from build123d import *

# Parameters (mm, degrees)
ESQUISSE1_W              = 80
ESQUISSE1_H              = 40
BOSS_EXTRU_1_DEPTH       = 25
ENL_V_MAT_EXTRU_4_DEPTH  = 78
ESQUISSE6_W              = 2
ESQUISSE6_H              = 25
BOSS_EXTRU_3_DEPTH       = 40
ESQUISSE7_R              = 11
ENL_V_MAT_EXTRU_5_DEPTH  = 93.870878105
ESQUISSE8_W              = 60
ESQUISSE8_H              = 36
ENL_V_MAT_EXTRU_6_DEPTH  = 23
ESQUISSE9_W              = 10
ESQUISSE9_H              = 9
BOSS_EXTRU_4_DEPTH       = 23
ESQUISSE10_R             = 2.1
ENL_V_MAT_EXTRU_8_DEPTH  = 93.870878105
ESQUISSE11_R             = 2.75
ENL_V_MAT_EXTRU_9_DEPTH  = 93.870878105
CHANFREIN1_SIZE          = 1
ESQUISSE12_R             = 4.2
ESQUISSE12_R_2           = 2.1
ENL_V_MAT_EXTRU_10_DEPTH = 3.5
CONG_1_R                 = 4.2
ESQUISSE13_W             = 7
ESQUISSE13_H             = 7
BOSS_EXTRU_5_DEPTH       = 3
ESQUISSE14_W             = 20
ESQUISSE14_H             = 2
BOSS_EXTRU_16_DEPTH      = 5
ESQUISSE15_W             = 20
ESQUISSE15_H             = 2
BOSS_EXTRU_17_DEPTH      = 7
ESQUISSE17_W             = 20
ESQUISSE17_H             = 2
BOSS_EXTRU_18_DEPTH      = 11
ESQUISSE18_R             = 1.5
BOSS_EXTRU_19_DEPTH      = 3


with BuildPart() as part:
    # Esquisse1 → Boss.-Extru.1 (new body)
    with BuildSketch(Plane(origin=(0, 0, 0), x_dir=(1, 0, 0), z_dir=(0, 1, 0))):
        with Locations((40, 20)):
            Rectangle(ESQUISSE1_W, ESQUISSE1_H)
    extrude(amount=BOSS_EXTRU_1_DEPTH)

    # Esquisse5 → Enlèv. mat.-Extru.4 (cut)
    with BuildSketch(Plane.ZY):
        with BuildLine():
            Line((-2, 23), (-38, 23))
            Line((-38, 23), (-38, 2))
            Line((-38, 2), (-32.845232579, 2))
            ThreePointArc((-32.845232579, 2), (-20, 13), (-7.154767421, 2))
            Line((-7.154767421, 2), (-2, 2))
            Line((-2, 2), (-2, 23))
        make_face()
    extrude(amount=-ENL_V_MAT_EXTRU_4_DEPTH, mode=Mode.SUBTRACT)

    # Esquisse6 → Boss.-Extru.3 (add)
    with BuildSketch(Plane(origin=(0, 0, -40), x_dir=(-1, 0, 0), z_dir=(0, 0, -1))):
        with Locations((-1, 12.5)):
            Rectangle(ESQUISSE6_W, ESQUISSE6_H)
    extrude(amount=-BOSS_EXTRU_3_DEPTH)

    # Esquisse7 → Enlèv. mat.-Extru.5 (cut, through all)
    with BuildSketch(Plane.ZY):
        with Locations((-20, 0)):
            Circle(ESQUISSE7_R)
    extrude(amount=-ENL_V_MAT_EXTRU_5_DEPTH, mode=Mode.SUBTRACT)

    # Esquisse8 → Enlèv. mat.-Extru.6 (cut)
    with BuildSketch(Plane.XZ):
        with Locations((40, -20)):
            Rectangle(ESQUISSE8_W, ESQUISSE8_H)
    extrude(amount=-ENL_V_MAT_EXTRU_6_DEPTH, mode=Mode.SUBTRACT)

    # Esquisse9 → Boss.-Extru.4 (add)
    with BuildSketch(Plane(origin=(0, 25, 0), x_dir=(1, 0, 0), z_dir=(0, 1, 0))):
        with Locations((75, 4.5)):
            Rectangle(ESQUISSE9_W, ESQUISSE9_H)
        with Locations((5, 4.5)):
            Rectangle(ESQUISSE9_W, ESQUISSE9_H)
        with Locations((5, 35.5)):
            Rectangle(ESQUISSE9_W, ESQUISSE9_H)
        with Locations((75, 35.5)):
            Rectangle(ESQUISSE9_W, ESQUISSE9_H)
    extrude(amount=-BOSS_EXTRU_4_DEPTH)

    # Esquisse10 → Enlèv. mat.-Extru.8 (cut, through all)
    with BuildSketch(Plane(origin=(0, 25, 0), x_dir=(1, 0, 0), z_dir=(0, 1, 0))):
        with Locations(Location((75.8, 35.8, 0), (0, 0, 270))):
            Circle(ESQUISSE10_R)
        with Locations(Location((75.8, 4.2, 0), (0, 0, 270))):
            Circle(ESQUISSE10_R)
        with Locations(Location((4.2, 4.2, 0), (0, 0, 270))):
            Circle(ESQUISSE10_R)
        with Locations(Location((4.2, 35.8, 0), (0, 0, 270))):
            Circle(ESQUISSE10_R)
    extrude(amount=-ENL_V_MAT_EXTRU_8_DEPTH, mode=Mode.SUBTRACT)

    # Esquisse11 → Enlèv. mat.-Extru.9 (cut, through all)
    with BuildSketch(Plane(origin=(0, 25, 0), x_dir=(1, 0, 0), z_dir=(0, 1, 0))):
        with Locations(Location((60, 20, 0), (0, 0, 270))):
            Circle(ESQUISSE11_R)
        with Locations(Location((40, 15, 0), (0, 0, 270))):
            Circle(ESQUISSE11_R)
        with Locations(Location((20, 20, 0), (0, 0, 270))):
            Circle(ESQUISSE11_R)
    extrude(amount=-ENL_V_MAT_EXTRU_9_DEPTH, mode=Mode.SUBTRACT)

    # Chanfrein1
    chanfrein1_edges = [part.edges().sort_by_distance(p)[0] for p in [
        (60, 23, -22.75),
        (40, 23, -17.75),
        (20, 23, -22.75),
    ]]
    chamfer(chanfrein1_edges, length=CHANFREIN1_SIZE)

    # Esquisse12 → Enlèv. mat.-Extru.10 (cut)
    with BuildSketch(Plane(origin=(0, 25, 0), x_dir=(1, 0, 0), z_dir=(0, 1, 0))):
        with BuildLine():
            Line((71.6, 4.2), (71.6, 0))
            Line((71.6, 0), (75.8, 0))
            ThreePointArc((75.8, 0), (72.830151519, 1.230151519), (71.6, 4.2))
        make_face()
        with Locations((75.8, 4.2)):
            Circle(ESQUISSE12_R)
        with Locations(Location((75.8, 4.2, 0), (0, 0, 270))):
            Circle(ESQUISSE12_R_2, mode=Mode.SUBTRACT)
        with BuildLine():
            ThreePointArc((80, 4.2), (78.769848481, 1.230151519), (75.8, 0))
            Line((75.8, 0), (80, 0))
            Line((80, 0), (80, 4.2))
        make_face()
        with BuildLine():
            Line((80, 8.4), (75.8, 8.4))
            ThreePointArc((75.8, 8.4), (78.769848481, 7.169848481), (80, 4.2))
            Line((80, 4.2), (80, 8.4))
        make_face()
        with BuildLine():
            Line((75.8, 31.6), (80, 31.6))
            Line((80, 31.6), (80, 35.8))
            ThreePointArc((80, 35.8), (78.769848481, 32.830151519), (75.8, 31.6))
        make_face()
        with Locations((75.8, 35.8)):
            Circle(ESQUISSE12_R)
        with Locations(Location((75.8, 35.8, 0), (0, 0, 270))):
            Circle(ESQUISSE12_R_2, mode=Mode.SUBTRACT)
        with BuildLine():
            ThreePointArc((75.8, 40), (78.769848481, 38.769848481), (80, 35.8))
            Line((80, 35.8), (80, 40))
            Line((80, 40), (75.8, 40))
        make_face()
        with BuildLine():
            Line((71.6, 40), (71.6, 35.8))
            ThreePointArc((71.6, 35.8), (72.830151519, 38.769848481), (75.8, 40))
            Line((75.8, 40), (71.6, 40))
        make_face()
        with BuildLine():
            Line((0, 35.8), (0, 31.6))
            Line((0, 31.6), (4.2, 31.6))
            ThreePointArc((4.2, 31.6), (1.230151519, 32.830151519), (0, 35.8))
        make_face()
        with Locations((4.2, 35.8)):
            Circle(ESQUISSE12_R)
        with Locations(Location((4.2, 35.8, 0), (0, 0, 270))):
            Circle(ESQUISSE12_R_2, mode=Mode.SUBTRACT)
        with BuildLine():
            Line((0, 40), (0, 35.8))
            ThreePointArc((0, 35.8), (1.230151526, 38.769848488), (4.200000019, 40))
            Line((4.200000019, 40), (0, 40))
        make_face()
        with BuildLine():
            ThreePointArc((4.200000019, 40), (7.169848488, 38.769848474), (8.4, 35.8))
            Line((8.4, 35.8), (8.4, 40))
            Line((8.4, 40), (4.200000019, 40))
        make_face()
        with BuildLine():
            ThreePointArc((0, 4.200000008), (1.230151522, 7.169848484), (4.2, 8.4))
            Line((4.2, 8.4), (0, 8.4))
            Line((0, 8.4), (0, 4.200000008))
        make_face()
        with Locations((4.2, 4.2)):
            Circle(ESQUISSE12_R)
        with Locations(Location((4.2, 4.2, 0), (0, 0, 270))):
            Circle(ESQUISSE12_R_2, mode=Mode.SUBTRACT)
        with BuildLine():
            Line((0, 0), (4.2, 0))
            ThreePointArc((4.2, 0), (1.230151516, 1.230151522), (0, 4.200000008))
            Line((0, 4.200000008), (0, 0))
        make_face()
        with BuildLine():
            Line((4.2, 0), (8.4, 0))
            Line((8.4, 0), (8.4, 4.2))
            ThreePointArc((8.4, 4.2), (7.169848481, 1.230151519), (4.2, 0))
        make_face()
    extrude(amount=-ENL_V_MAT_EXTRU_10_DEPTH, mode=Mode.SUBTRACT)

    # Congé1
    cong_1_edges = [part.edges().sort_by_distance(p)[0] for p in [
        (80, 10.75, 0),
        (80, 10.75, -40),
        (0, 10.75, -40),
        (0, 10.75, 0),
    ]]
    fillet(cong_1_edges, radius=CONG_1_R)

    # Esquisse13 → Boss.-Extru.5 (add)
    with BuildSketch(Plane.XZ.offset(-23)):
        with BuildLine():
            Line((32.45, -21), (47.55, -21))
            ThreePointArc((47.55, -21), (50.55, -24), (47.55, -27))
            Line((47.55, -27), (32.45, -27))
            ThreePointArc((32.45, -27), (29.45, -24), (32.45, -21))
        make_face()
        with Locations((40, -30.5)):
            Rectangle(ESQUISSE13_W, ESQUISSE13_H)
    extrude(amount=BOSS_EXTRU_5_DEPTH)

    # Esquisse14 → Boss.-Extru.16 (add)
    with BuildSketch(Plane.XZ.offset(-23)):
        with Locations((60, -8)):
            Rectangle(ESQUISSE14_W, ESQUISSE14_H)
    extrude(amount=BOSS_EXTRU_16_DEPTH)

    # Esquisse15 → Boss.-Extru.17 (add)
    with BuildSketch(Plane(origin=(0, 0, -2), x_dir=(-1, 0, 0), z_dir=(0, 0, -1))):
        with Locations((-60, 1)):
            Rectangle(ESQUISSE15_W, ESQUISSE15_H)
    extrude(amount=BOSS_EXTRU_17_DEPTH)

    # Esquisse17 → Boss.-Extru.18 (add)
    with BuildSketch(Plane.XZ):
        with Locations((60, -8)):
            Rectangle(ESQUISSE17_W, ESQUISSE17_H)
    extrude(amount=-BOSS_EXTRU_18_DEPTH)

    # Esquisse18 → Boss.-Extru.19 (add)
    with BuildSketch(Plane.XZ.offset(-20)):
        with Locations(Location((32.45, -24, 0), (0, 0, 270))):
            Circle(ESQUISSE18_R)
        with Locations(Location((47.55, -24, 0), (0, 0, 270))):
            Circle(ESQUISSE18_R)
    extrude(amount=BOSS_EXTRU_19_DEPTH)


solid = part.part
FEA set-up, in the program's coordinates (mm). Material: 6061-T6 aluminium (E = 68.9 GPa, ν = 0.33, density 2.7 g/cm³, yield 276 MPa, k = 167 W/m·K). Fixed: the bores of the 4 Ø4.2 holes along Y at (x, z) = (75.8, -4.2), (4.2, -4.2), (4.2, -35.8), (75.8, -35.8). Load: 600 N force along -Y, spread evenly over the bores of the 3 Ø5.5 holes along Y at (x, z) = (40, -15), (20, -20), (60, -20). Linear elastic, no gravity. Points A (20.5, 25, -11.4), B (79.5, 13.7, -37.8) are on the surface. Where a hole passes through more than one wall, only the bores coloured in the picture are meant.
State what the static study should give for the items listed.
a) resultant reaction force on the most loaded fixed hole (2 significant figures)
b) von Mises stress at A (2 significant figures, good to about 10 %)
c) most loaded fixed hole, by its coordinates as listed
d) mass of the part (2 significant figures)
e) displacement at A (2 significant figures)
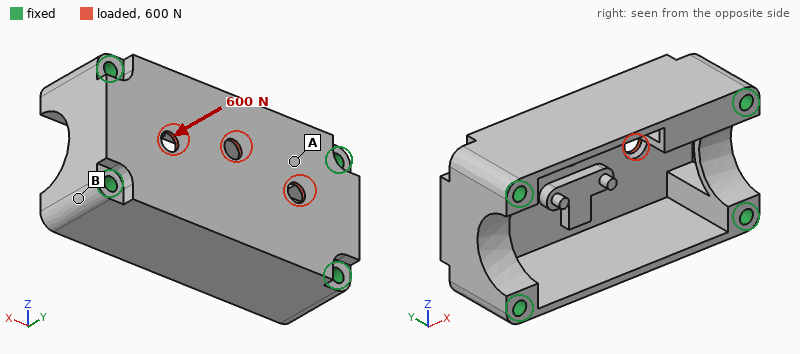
280 N
23 MPa
(75.8, -4.2)
57 g
41 µm
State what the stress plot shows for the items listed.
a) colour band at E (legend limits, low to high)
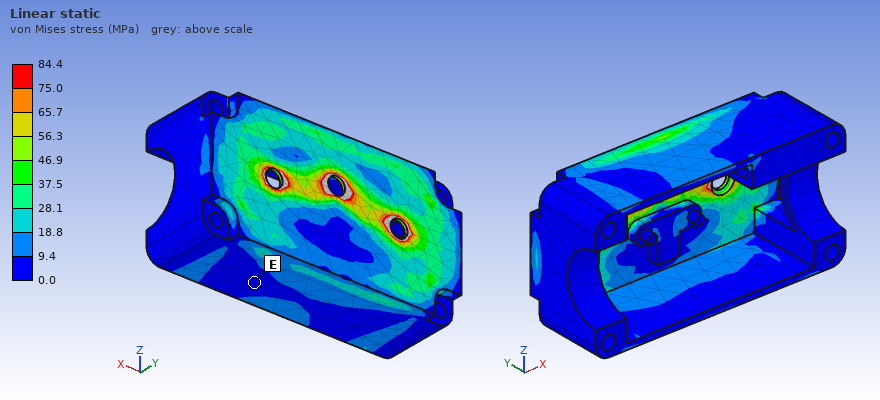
0.0 to 9.4 MPa
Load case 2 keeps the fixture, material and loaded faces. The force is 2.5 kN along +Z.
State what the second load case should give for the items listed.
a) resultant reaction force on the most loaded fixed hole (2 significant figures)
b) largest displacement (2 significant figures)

740 N
27 µm
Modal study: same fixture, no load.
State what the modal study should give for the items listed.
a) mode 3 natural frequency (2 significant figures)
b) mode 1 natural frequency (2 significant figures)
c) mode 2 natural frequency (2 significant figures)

6900 Hz
4100 Hz
5600 Hz
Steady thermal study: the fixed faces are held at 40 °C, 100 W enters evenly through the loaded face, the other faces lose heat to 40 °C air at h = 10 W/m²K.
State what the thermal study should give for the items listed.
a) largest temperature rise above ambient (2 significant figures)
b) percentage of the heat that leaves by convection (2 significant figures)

75 K
3.3 %
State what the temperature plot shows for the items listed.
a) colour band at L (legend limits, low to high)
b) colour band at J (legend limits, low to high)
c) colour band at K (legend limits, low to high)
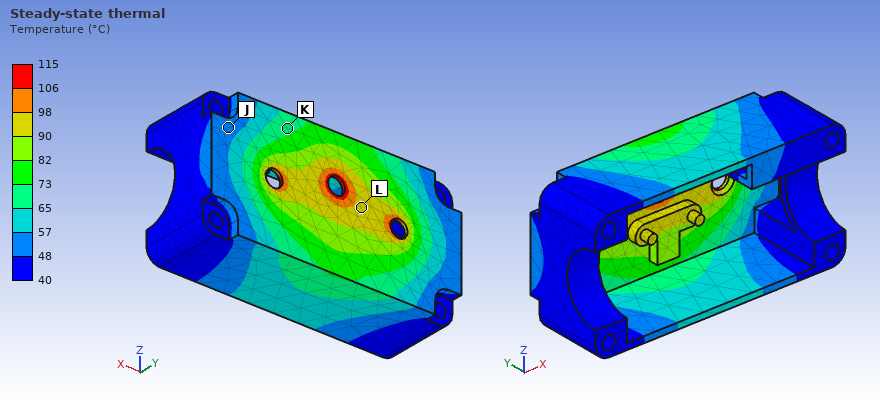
90 to 98 °C
48 to 57 °C
65 to 73 °C
